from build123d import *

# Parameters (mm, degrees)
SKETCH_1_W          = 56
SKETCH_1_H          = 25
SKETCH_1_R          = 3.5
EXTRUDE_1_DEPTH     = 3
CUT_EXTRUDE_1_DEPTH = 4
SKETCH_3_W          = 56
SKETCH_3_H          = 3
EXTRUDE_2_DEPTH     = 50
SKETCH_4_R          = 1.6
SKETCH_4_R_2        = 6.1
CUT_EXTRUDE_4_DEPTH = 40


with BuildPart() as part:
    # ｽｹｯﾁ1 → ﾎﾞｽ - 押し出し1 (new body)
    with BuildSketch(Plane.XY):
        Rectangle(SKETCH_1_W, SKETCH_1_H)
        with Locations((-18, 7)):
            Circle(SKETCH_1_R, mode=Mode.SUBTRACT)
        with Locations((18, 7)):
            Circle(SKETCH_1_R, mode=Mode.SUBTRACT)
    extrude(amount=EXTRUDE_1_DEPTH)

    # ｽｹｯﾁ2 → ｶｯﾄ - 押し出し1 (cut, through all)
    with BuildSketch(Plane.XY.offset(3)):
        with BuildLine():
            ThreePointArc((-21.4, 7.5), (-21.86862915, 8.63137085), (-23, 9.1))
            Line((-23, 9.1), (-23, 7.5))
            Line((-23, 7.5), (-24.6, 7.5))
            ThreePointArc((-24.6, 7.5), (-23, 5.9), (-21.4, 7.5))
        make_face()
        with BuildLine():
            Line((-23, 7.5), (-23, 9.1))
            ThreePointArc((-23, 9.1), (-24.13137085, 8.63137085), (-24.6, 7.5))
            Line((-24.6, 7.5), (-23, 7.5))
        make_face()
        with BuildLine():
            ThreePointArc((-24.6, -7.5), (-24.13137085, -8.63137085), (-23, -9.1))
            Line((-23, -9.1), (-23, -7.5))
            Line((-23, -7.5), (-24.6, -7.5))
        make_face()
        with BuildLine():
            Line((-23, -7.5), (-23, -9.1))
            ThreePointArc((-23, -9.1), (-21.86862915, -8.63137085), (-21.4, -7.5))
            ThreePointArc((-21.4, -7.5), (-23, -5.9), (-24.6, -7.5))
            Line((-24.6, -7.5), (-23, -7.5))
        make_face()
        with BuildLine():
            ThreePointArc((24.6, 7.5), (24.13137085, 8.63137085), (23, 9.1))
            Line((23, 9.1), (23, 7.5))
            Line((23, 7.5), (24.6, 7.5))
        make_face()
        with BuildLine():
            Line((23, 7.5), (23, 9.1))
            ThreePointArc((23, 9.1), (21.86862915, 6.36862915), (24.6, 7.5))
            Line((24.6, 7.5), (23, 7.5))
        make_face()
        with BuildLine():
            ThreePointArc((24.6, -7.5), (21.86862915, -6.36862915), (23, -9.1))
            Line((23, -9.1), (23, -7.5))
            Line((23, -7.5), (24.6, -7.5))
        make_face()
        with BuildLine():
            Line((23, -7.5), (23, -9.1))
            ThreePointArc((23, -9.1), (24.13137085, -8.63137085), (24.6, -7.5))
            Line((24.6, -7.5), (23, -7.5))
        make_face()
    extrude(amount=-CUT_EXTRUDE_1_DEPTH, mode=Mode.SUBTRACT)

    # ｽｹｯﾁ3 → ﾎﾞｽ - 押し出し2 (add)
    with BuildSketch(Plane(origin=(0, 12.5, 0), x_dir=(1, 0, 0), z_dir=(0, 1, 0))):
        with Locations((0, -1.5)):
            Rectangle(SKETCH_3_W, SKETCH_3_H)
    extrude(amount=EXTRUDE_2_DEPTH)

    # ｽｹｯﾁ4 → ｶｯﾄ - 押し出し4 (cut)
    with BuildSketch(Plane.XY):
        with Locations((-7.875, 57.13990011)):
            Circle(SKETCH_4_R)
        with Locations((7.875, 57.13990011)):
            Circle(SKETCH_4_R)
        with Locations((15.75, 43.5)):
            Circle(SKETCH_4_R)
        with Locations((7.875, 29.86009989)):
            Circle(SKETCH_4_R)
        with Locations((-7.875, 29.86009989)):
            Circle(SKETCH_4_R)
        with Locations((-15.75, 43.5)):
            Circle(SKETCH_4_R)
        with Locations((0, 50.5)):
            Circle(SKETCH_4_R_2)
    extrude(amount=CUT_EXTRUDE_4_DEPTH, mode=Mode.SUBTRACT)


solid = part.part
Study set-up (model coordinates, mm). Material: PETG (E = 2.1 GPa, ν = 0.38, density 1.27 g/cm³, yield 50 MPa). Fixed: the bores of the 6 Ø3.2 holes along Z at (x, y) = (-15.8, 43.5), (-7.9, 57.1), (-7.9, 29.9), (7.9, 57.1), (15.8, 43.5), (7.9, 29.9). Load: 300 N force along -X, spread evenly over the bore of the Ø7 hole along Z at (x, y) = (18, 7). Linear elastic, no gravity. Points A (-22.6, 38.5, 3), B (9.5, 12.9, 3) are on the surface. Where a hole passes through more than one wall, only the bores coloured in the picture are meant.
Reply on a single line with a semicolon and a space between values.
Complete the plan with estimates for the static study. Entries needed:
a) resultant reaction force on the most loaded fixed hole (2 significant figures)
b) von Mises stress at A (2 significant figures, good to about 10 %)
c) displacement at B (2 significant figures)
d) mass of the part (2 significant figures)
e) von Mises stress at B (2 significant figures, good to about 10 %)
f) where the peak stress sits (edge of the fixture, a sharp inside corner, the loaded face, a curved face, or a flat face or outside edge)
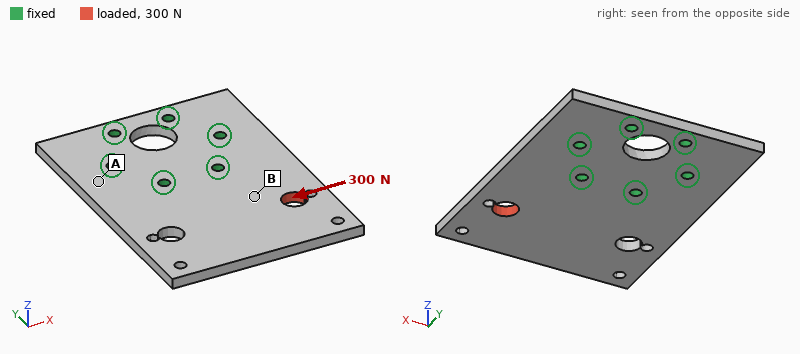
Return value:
200 N; 2.5 MPa; 0.092 mm; 15 g; 5.1 MPa; the loaded face
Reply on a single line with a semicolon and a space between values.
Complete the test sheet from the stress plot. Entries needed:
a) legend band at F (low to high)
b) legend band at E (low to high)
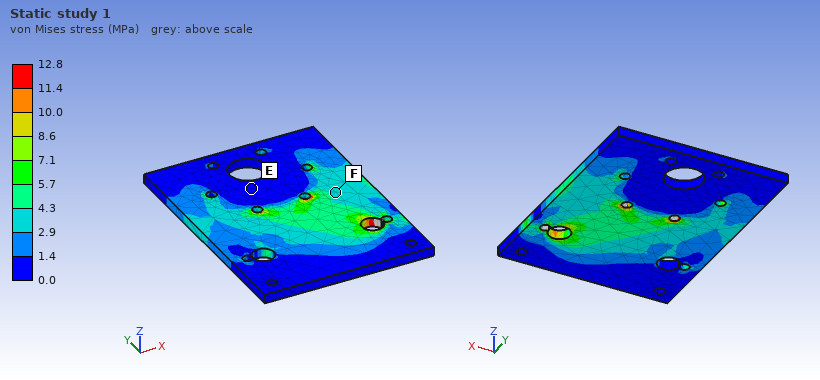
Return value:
2.9 to 4.3 MPa; 0.0 to 1.4 MPa
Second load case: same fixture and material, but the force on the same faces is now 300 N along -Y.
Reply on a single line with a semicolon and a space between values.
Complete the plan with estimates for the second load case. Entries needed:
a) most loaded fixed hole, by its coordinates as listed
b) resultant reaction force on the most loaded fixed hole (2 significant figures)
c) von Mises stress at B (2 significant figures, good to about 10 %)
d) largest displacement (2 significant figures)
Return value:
(7.9, 29.9); 170 N; 3.9 MPa; 0.15 mm
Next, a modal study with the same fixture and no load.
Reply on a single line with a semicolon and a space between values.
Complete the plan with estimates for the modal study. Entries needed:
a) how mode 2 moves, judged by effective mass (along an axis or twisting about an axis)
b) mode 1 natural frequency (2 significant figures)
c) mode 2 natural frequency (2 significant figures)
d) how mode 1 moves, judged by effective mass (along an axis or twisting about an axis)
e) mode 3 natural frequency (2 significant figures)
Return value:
twisting about Y; 340 Hz; 590 Hz; along Z; 1400 Hz
